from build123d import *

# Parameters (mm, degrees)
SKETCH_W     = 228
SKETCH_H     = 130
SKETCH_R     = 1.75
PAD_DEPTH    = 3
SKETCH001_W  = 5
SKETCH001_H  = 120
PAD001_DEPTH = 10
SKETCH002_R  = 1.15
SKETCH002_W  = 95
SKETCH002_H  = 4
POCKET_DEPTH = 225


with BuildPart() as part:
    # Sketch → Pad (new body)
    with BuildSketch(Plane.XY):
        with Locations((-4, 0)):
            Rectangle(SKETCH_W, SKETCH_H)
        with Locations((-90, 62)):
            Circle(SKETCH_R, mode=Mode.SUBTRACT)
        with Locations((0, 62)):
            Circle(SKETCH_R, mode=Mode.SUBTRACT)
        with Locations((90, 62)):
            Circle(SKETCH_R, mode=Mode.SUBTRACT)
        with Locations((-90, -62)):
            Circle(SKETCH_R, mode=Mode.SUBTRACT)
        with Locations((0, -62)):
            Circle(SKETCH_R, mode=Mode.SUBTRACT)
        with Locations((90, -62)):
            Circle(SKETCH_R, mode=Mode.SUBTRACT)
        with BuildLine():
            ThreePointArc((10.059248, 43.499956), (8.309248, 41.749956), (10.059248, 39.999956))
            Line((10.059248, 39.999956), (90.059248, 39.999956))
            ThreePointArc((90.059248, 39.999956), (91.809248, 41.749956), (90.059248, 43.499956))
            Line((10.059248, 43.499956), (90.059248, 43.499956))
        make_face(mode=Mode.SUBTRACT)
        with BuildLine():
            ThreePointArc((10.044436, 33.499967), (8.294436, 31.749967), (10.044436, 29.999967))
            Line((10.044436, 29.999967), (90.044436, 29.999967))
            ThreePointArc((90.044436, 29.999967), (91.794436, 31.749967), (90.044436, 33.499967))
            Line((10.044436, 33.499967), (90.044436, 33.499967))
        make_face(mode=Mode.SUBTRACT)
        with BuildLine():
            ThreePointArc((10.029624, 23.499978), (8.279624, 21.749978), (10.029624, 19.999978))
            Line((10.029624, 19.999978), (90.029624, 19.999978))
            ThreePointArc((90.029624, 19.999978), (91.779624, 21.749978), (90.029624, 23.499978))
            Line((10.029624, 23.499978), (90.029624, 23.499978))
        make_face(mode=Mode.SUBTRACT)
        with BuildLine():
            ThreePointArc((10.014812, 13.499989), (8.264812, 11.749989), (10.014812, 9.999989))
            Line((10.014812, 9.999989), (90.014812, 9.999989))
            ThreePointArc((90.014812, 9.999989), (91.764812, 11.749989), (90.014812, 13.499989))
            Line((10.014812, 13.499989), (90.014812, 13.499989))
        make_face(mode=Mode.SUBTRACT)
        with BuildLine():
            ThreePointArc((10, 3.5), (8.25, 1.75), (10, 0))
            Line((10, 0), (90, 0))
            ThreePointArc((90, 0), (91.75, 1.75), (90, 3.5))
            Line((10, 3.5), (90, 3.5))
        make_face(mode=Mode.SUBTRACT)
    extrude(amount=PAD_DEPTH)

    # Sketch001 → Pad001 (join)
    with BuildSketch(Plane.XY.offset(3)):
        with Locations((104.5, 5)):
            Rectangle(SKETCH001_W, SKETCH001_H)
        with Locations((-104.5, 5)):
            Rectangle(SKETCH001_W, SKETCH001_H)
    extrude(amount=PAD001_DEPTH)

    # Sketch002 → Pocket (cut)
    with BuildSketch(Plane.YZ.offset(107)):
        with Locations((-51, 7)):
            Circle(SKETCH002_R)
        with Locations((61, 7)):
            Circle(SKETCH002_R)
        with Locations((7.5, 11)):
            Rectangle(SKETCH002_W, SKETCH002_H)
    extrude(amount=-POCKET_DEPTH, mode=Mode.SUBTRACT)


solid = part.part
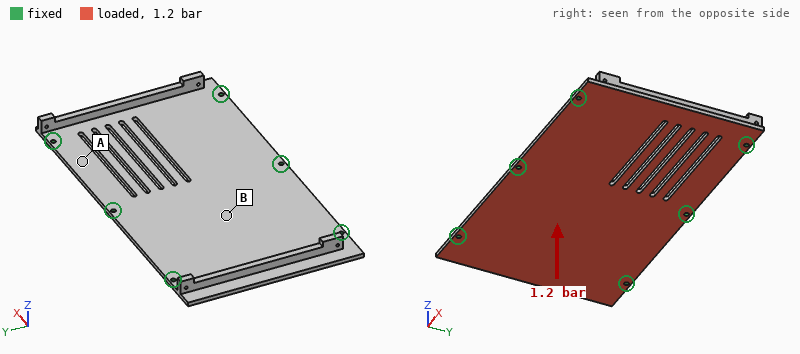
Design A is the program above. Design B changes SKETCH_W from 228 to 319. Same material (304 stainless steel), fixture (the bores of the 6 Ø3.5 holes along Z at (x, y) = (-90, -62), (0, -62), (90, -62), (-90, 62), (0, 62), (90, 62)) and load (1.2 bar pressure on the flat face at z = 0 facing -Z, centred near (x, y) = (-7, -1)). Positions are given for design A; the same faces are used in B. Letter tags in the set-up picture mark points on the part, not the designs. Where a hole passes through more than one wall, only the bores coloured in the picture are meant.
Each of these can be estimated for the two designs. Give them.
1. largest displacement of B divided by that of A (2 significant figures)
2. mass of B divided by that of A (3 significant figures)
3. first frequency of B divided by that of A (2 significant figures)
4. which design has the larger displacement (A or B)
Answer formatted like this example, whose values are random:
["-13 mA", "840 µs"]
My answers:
["3.5", "1.38", "0.49", "B"]
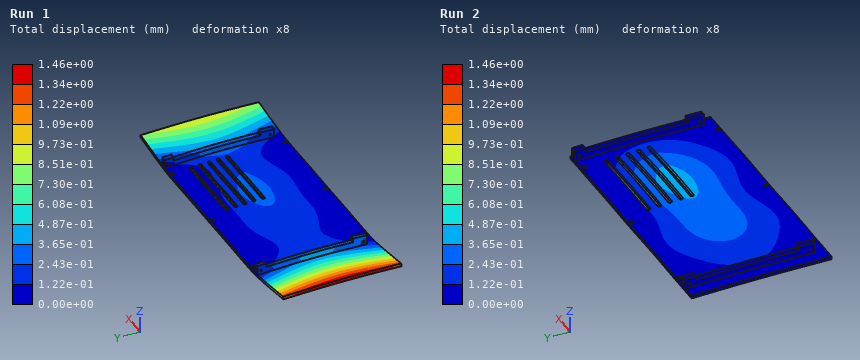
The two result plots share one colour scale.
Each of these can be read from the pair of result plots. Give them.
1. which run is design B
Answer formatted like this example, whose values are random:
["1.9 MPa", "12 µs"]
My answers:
["Run 1"]
